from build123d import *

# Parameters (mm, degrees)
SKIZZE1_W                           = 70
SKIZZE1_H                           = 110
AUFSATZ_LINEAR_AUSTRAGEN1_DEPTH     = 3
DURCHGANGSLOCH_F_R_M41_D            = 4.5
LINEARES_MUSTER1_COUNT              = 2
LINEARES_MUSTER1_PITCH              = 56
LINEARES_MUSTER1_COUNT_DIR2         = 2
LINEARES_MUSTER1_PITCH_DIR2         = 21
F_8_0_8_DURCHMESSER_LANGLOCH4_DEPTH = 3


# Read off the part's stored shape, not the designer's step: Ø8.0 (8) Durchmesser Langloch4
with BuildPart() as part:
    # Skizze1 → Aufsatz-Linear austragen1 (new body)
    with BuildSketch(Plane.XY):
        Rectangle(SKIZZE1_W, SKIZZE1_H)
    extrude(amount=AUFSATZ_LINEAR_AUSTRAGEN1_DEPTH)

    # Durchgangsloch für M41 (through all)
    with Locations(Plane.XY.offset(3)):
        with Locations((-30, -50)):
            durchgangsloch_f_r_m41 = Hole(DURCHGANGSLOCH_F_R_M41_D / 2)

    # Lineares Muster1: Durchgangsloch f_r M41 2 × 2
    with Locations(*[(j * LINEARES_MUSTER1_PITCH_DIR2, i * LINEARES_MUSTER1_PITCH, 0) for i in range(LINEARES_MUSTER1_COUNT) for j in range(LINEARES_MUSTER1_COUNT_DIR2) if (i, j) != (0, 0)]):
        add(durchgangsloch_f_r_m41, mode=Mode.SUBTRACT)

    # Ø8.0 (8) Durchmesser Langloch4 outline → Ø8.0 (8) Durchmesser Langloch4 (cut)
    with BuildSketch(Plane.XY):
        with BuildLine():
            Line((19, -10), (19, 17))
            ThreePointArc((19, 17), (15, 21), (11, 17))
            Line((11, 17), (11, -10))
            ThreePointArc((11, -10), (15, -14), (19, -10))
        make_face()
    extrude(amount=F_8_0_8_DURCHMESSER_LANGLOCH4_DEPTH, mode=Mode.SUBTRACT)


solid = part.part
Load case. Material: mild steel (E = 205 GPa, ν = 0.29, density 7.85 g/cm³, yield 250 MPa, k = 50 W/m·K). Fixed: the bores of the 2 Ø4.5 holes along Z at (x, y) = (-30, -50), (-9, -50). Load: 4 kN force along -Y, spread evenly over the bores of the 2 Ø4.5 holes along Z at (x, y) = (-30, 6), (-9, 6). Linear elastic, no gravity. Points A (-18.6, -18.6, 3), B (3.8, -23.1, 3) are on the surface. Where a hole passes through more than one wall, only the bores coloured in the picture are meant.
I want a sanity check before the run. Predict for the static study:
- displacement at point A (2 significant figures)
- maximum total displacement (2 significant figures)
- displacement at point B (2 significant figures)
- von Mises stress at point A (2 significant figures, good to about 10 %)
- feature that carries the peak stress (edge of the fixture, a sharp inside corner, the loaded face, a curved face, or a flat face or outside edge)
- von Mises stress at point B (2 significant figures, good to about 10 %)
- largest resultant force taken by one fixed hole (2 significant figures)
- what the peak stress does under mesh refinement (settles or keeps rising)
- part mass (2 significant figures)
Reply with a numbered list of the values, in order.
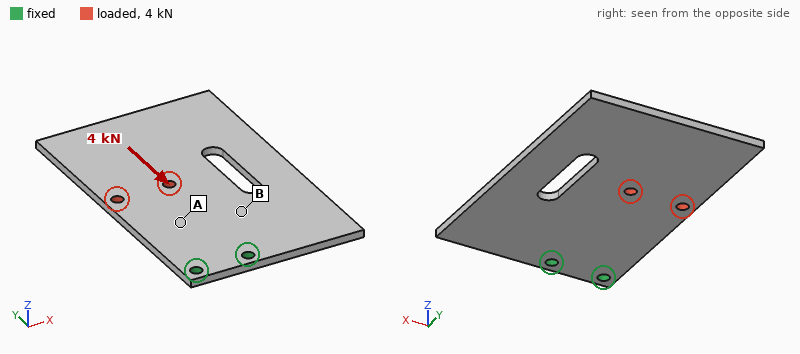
1. 6.4 µm
2. 22 µm
3. 3.3 µm
4. 36 MPa
5. edge of the fixture
6. 12 MPa
7. 2.0 kN
8. keeps rising
9. 170 g
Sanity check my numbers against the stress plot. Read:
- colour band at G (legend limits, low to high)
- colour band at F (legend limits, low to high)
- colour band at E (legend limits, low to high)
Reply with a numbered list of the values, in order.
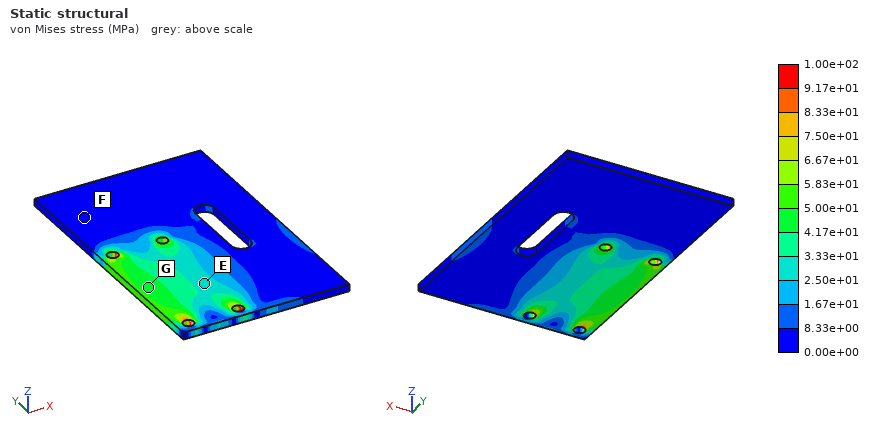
1. 4.17e+01 to 5.00e+01 MPa
2. 0.00e+00 to 8.33e+00 MPa
3. 2.50e+01 to 3.33e+01 MPa
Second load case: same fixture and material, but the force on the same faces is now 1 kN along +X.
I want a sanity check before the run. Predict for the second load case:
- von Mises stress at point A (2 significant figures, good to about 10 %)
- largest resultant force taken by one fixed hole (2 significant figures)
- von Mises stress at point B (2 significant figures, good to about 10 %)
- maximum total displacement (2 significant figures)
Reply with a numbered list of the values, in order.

1. 21 MPa
2. 2.4 kN
3. 15 MPa
4. 64 µm
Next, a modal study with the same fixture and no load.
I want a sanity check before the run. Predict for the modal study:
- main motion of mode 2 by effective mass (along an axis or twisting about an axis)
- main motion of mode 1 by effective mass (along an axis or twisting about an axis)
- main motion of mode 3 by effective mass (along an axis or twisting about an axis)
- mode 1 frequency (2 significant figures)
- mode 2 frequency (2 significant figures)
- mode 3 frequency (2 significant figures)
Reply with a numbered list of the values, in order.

1. twisting about Y
2. along Z
3. along Z
4. 200 Hz
5. 590 Hz
6. 1200 Hz
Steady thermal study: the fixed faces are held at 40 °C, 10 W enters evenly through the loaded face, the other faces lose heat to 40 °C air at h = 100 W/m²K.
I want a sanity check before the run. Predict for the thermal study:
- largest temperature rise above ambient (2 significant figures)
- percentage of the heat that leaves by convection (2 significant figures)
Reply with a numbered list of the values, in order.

1. 28 K
2. 90 %
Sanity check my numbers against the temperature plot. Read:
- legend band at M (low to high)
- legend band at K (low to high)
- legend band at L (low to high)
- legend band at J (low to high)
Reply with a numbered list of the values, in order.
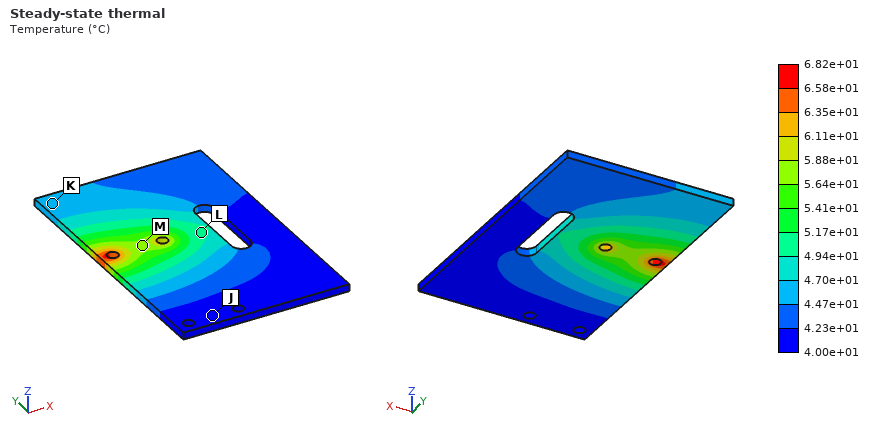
1. 5.64e+01 to 5.88e+01 °C
2. 4.47e+01 to 4.70e+01 °C
3. 4.94e+01 to 5.17e+01 °C
4. 4.00e+01 to 4.23e+01 °C
